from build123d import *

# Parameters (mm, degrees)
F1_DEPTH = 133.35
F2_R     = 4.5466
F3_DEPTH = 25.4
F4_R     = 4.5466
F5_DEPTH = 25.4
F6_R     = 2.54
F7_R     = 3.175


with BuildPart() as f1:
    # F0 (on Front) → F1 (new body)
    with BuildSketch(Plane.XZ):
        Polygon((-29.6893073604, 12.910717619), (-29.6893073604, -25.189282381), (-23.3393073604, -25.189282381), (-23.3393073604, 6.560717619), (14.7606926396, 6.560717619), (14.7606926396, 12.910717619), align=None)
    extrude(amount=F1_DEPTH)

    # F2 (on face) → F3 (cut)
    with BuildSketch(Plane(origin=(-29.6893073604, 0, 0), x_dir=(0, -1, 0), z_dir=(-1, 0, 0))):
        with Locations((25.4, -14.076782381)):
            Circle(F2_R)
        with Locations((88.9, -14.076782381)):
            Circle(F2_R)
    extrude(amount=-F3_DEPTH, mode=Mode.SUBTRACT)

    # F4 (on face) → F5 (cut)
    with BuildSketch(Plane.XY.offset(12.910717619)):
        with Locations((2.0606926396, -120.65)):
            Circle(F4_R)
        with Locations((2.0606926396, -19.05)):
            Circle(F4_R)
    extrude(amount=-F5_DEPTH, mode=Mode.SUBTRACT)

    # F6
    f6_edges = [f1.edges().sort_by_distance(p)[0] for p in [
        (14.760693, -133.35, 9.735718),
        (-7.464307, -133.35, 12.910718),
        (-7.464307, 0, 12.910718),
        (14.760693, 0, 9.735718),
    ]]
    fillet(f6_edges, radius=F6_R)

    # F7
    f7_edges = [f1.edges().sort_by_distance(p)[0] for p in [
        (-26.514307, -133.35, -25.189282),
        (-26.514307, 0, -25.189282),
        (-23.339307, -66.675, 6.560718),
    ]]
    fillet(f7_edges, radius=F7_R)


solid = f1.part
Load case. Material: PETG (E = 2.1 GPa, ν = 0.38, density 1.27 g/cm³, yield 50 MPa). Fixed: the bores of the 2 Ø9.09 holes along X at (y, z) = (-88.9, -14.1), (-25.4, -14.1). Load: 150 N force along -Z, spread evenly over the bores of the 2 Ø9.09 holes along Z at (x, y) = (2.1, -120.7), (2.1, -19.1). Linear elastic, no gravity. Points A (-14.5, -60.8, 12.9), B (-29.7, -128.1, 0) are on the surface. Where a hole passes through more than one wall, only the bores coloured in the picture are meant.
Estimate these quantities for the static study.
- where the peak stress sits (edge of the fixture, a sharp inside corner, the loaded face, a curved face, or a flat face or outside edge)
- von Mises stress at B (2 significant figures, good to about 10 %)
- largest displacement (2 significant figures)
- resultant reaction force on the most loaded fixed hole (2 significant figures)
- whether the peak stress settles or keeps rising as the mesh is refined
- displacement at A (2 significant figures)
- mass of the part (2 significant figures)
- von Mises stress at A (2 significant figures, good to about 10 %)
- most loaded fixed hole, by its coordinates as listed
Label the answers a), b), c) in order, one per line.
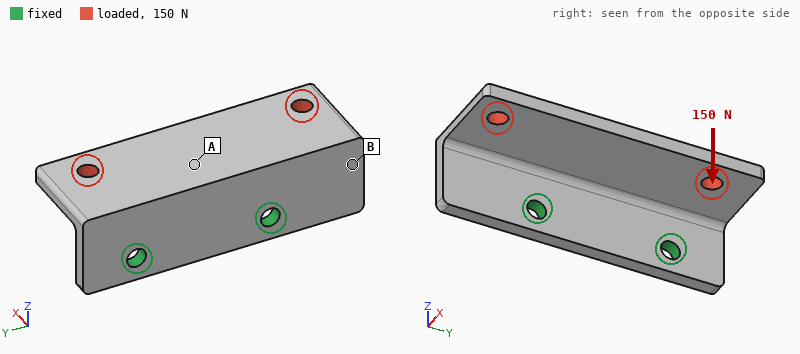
a) edge of the fixture
b) 3.8 MPa
c) 1.3 mm
d) 100 N
e) keeps rising
f) 0.34 mm
g) 80 g
h) 2.1 MPa
i) (-88.9, -14.1)
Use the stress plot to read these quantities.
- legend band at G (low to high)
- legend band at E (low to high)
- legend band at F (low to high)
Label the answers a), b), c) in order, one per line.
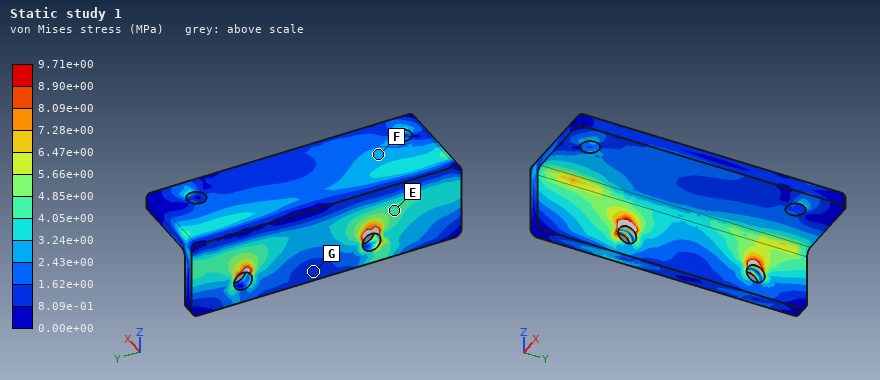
a) 8.09e-01 to 1.62e+00 MPa
b) 4.05e+00 to 4.85e+00 MPa
c) 2.43e+00 to 3.24e+00 MPa
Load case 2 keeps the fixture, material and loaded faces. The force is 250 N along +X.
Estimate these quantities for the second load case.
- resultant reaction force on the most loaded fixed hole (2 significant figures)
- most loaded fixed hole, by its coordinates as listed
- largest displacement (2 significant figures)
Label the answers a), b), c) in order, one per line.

a) 170 N
b) (-88.9, -14.1)
c) 0.83 mm
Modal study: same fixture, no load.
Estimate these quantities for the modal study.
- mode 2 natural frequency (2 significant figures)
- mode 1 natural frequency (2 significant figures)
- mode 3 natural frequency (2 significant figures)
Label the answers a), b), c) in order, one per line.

a) 550 Hz
b) 390 Hz
c) 890 Hz
